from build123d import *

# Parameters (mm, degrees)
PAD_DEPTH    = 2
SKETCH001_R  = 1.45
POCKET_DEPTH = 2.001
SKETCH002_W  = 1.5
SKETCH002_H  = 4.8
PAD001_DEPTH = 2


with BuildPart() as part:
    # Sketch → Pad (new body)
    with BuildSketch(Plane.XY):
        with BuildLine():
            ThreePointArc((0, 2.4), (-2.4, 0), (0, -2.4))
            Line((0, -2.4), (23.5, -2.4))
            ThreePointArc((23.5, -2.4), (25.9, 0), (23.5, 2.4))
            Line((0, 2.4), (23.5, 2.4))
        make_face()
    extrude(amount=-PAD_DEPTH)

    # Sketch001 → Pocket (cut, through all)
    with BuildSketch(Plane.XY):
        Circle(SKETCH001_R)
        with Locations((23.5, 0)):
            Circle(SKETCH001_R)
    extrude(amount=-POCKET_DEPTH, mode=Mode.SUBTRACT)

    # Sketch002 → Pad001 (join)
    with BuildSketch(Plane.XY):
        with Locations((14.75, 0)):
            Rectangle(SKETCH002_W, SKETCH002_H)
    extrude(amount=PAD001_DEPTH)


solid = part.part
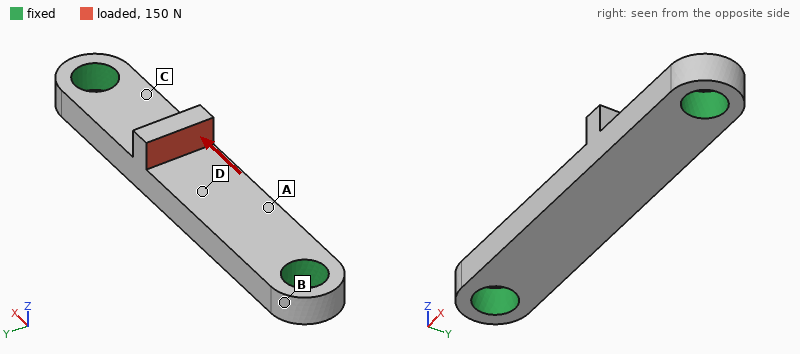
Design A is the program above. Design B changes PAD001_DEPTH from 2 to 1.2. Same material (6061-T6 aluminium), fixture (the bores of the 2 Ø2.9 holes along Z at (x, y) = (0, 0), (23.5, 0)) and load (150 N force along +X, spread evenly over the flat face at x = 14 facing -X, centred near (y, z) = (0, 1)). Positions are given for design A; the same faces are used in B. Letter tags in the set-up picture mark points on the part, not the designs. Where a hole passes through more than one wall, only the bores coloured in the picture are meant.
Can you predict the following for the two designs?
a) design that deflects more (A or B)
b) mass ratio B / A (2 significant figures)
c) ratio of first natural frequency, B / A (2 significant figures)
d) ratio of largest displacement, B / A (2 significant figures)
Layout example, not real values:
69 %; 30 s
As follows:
A; 0.98; 1.0; 0.63
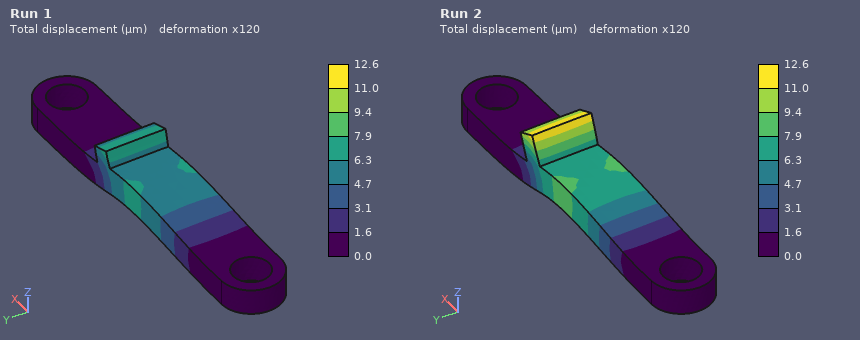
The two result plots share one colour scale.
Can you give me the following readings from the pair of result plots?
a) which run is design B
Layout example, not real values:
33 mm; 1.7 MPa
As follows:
Run 1
